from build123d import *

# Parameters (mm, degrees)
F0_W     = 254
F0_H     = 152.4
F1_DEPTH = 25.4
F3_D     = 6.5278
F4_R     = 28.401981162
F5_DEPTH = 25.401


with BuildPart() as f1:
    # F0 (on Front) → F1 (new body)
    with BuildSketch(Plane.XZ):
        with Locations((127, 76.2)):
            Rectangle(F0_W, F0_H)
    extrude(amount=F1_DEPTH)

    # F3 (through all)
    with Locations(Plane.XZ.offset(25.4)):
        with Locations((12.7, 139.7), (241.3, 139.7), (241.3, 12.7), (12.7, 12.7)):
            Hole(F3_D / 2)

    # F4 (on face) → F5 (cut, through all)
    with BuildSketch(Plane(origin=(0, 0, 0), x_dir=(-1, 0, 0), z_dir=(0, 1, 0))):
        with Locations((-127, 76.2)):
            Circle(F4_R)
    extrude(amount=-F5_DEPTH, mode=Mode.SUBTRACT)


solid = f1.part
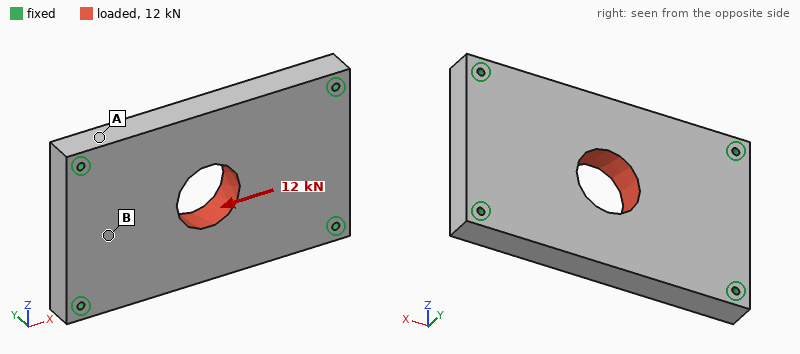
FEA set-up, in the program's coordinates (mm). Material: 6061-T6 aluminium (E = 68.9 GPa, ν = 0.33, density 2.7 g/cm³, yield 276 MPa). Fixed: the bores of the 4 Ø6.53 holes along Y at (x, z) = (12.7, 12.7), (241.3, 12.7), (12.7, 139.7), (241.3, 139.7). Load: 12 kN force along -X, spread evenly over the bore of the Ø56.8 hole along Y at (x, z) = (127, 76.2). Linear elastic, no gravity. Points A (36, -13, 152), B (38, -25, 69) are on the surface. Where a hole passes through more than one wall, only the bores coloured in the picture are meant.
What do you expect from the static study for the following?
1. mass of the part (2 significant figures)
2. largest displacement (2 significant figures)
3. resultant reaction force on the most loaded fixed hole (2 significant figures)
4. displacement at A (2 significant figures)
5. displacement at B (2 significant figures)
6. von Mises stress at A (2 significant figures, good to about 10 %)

2.5 kg
4.7 µm
3.2 kN
1.3 µm
3.2 µm
2.9 MPa
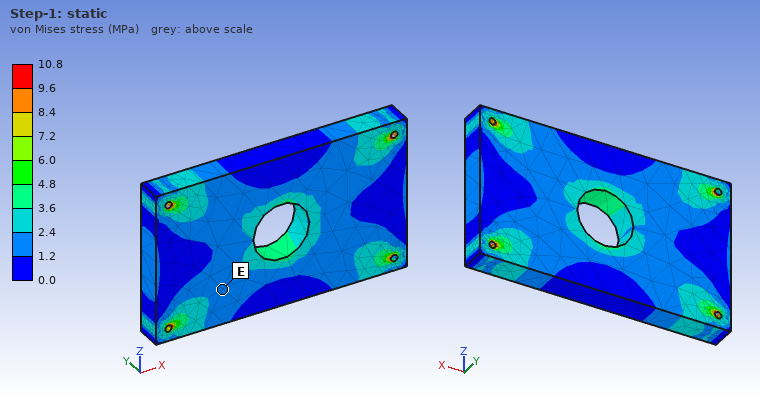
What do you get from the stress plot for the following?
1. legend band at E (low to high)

1.2 to 2.4 MPa
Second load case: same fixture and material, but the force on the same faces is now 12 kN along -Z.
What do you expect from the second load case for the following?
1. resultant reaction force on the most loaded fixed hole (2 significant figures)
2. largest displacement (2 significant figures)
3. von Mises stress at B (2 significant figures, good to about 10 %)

3.9 kN
10 µm
3.1 MPa
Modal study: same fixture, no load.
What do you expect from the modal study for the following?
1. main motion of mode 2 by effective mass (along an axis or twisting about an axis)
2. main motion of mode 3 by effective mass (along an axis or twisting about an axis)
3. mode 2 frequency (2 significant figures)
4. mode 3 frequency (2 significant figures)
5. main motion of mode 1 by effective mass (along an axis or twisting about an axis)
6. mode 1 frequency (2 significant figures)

twisting about X
twisting about Z
2900 Hz
4300 Hz
along Y
1800 Hz
